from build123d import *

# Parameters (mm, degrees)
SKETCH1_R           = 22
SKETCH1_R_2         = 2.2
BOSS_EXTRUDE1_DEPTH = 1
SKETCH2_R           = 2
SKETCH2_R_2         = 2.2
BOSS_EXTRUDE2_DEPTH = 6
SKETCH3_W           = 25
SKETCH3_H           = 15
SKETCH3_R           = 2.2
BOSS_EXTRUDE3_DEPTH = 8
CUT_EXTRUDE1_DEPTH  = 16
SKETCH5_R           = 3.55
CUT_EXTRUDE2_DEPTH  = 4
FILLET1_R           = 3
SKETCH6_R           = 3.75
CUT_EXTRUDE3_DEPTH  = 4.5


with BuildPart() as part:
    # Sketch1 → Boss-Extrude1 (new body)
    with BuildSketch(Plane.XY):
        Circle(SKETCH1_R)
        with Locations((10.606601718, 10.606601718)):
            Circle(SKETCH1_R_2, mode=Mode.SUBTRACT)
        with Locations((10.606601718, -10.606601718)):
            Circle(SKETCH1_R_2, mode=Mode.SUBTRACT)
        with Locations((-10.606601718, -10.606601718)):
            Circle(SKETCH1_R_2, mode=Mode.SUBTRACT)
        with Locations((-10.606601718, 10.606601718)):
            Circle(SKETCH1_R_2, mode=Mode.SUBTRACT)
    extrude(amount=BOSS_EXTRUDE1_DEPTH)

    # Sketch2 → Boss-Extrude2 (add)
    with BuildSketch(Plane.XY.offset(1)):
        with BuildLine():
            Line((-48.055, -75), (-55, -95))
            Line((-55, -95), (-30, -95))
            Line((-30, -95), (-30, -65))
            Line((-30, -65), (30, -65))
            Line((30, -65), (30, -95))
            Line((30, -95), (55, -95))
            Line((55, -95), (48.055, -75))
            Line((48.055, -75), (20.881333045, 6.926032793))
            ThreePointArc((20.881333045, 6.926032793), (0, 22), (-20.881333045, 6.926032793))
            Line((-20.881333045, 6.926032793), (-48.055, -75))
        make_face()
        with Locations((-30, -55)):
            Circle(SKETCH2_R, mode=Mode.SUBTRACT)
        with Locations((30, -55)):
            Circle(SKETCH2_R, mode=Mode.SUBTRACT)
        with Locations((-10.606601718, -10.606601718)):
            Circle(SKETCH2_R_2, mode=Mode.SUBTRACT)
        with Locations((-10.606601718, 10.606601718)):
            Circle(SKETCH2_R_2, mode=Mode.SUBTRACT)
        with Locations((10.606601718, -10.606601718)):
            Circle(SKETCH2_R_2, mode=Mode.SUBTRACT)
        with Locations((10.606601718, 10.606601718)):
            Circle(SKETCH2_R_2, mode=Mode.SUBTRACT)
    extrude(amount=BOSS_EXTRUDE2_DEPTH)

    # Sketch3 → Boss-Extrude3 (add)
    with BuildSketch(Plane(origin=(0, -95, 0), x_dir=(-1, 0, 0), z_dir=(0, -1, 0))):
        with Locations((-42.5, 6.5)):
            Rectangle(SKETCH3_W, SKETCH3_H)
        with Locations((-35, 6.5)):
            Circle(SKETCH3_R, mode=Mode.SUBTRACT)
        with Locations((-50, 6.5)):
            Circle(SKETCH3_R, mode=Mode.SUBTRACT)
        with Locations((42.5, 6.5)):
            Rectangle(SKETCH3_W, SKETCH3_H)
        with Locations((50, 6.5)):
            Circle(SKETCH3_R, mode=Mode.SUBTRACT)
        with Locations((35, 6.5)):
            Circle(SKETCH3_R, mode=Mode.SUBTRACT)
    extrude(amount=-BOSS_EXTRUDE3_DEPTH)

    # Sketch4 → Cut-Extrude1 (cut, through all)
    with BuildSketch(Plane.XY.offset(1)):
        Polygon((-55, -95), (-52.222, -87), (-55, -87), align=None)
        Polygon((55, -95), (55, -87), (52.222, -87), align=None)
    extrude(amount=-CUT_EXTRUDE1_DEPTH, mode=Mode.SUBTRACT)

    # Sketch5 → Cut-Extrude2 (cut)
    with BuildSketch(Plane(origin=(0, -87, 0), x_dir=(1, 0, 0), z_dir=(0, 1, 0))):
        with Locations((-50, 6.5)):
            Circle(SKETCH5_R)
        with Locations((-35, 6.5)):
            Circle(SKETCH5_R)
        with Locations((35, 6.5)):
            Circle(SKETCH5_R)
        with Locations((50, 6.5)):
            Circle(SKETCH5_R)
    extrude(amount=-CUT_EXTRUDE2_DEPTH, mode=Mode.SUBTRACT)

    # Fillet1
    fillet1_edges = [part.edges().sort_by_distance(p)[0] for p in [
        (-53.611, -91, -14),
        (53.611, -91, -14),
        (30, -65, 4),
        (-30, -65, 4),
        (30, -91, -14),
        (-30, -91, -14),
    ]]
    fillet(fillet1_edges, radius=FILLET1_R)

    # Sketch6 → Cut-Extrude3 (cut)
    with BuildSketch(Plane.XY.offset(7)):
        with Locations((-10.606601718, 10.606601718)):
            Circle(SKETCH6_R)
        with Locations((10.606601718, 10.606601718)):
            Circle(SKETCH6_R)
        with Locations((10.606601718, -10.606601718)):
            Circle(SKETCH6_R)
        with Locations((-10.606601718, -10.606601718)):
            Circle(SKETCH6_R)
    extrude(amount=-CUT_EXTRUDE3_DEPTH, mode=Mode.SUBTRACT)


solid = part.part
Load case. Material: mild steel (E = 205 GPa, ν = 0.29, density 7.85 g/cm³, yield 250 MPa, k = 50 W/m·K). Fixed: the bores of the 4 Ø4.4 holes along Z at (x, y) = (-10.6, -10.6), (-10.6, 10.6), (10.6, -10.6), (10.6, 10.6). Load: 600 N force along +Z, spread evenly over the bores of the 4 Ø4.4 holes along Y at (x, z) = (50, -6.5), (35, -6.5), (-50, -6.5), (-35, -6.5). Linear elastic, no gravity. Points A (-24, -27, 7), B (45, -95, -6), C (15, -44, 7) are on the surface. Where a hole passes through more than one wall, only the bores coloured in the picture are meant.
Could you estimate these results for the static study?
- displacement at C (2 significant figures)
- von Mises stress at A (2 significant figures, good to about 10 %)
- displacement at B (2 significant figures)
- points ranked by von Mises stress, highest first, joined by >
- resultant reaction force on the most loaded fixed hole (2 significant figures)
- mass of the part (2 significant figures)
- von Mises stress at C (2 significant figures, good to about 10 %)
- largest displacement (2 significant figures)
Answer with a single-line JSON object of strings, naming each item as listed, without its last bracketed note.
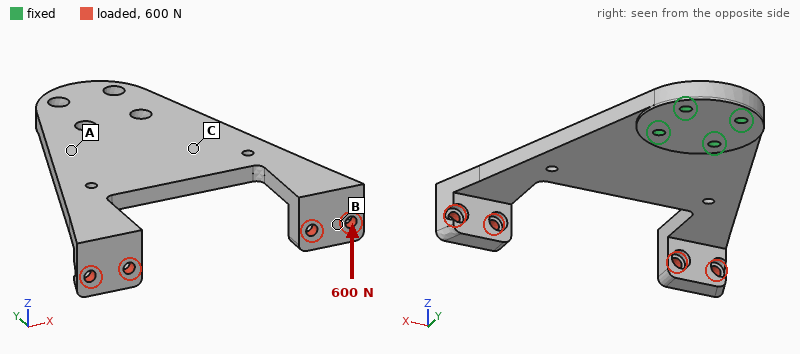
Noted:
{"displacement at C": "0.12 mm", "von Mises stress at A": "100 MPa", "displacement at B": "0.65 mm", "points ranked by von Mises stress, highest first, joined by >": "A > C > B", "resultant reaction force on the most loaded fixed hole": "2.0 kN", "mass of the part": "340 g", "von Mises stress at C": "57 MPa", "largest displacement": "0.69 mm"}
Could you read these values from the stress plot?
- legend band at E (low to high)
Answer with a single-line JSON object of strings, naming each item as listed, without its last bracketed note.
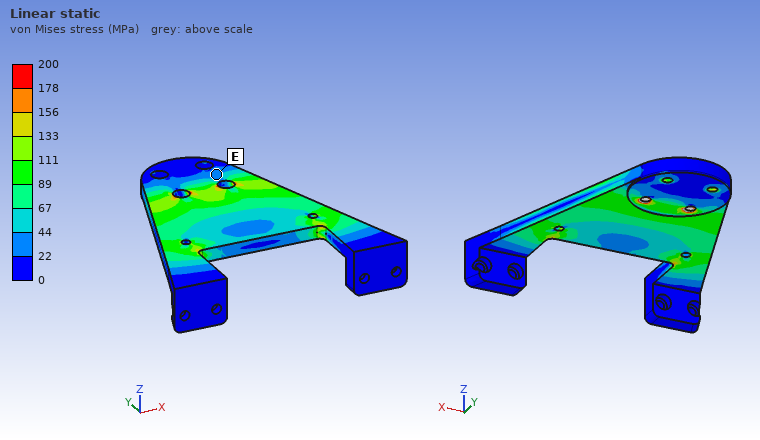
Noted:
{"legend band at E": "22 to 44 MPa"}
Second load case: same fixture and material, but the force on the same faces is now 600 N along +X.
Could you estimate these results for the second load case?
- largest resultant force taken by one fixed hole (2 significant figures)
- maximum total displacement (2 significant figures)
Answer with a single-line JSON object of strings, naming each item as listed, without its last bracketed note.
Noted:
{"largest resultant force taken by one fixed hole": "1.1 kN", "maximum total displacement": "0.11 mm"}
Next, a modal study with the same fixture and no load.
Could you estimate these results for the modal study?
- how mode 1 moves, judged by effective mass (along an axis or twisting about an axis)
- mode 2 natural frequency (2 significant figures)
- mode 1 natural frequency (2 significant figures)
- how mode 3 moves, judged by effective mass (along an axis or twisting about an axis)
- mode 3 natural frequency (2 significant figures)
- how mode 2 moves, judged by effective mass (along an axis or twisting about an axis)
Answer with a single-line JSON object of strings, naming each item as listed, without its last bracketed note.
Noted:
{"how mode 1 moves, judged by effective mass": "along Z", "mode 2 natural frequency": "710 Hz", "mode 1 natural frequency": "540 Hz", "how mode 3 moves, judged by effective mass": "along X", "mode 3 natural frequency": "2200 Hz", "how mode 2 moves, judged by effective mass": "twisting about Y"}
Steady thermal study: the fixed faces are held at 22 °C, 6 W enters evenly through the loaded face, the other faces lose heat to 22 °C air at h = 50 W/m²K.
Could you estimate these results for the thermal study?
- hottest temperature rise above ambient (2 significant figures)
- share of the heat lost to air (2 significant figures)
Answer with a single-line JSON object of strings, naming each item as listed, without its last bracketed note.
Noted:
{"hottest temperature rise above ambient": "18 K", "share of the heat lost to air": "81 %"}
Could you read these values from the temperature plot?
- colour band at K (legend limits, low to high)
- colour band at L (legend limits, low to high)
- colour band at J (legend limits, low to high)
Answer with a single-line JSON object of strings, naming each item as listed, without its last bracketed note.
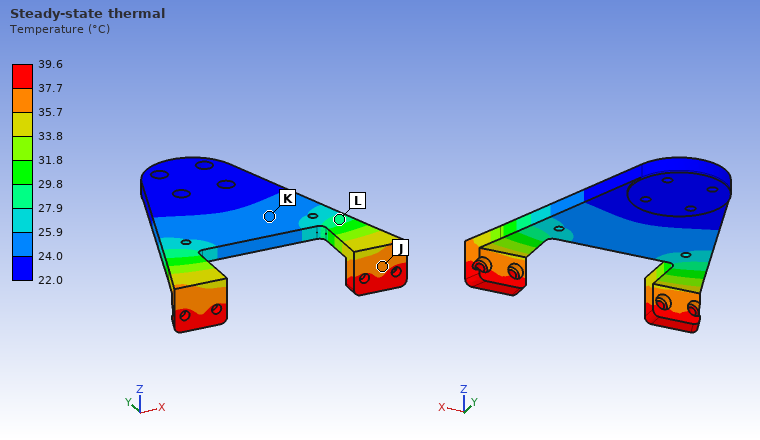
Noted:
{"colour band at K": "24.0 to 25.9 °C", "colour band at L": "27.9 to 29.8 °C", "colour band at J": "35.7 to 37.7 °C"}
